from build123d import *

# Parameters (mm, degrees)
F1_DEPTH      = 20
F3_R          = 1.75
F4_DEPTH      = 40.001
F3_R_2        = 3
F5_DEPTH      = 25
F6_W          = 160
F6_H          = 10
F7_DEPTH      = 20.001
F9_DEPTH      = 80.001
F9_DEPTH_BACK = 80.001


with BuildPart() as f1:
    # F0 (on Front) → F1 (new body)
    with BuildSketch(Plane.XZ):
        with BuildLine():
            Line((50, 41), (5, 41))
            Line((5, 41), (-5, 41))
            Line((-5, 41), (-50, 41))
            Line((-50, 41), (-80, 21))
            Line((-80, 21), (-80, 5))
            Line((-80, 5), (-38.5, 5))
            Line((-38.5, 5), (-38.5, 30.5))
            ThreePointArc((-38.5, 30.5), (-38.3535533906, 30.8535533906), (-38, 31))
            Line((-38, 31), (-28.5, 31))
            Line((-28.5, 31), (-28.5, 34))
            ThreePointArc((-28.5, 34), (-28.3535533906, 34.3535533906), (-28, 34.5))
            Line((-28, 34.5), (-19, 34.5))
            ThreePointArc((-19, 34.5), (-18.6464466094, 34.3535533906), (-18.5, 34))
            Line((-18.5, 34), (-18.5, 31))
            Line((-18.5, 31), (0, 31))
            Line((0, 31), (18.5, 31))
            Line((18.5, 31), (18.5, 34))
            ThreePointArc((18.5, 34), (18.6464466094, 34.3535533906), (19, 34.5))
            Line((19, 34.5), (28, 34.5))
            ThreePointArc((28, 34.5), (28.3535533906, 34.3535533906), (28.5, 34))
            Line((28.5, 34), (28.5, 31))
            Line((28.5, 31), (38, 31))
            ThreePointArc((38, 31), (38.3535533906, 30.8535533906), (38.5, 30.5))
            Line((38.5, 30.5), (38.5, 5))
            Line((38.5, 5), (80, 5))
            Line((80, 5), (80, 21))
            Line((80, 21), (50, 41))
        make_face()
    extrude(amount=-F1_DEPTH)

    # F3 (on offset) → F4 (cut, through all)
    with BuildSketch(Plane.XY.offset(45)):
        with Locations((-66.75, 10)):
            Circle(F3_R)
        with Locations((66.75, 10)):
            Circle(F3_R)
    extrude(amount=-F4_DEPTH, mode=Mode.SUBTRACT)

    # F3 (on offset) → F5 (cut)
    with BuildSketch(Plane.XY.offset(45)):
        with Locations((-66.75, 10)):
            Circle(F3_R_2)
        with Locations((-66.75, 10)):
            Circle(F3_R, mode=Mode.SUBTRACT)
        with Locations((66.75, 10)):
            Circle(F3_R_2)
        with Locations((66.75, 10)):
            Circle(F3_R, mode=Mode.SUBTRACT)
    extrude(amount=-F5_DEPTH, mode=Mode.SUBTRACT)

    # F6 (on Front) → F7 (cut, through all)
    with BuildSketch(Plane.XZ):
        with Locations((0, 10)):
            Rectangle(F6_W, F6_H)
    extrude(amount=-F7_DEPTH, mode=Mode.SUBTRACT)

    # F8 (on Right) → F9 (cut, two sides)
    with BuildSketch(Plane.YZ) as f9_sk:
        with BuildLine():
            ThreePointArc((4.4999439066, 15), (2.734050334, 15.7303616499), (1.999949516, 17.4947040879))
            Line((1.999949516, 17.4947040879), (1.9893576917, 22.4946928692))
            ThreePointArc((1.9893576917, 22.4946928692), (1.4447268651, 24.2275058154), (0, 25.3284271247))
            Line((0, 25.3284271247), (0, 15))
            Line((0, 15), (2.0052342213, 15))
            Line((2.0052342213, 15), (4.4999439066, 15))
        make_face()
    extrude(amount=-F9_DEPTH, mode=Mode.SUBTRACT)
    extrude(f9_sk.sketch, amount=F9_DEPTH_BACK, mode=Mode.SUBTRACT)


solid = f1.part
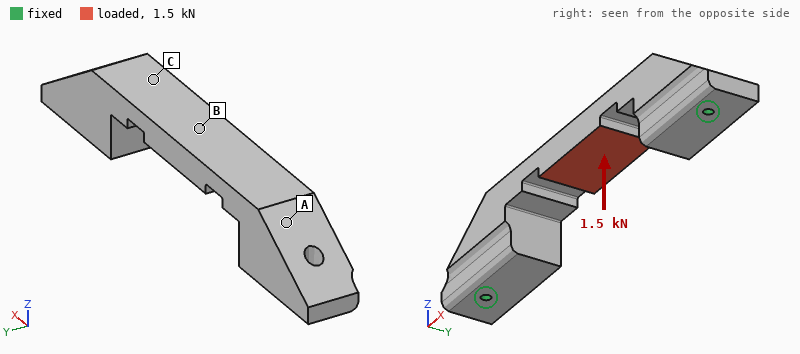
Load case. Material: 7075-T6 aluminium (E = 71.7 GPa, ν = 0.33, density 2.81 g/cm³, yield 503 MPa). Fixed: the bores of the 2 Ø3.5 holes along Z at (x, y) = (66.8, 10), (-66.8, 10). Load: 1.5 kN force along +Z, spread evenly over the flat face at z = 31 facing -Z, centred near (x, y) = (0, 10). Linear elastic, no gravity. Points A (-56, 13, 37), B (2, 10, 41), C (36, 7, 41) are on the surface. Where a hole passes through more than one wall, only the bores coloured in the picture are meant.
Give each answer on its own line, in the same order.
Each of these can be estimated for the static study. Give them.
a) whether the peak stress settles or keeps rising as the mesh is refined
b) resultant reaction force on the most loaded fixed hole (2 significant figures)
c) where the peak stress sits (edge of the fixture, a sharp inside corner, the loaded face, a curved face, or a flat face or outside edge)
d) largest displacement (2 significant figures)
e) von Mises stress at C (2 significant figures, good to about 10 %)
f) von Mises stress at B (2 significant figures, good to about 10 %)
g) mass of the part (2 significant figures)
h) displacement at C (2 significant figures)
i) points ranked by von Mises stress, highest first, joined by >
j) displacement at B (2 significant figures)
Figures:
keeps rising
1.7 kN
edge of the fixture
70 µm
14 MPa
46 MPa
120 g
23 µm
B > C > A
67 µm
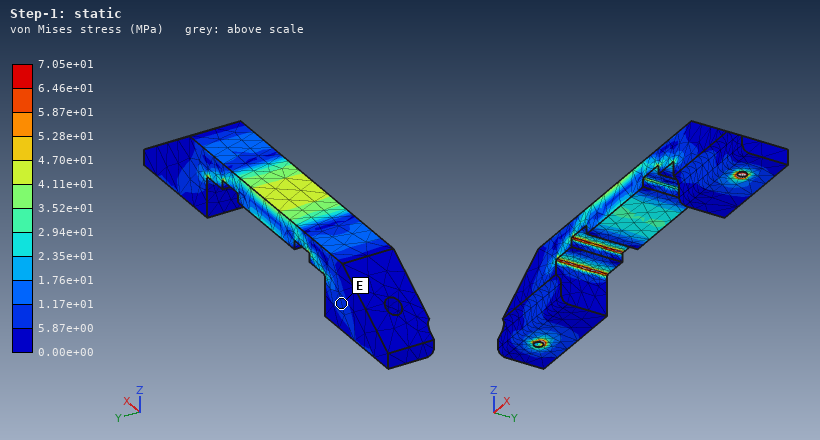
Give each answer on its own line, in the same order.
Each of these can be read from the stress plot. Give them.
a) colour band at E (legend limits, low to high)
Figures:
5.87e+00 to 1.17e+01 MPa
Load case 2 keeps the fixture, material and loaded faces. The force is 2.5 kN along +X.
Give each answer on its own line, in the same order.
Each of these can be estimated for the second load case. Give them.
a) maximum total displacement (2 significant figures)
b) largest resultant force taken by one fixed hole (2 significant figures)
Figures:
94 µm
1.3 kN
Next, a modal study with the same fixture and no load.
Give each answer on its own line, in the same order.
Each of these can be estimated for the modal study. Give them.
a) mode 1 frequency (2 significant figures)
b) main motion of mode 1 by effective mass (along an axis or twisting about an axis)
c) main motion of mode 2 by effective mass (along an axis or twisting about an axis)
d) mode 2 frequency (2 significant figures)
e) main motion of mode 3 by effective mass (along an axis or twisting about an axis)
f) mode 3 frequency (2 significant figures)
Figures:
2200 Hz
along Y
along X
3400 Hz
along Z
4600 Hz
